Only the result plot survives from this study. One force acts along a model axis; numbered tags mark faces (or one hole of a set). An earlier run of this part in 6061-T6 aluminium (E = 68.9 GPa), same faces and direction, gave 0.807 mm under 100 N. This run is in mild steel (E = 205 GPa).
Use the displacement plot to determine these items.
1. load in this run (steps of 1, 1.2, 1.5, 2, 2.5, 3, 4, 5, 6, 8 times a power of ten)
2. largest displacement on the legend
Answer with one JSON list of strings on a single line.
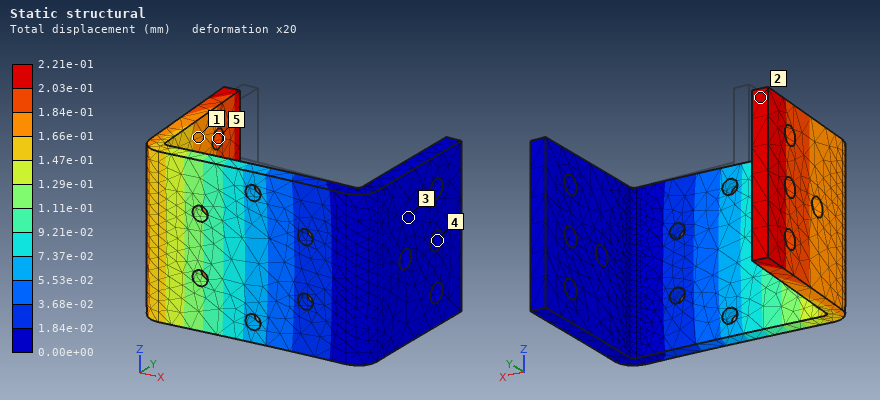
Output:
["80 N", "2.21e-01 mm"]
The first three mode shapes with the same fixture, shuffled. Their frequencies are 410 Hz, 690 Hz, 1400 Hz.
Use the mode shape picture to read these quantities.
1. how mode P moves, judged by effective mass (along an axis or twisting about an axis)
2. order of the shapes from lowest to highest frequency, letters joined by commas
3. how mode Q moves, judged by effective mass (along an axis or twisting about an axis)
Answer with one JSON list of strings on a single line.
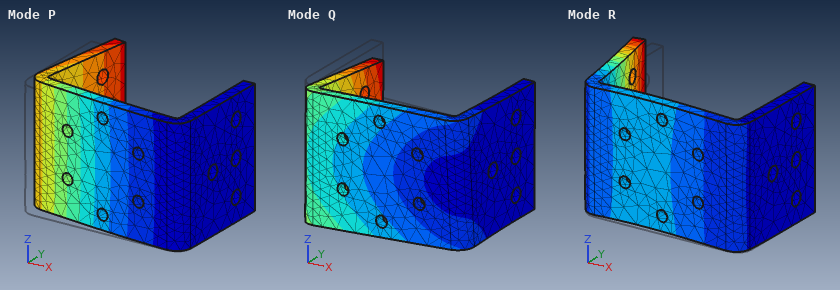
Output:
["along Y", "P, Q, R", "along Z"]
